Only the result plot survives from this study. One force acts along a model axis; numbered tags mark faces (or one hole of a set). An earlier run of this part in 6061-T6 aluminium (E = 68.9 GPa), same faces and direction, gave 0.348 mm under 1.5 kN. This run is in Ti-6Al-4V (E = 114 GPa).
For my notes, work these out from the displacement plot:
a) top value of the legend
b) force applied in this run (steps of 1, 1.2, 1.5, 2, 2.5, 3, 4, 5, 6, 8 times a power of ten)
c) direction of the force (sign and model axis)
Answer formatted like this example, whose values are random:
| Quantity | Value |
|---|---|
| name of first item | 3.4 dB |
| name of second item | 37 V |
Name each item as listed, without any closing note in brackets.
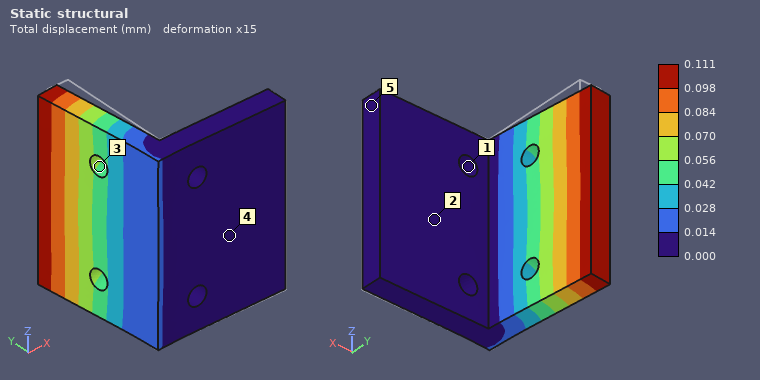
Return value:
| Quantity | Value |
|---|---|
| top value of the legend | 0.111 mm |
| force applied in this run | 800 N |
| direction of the force | -X |
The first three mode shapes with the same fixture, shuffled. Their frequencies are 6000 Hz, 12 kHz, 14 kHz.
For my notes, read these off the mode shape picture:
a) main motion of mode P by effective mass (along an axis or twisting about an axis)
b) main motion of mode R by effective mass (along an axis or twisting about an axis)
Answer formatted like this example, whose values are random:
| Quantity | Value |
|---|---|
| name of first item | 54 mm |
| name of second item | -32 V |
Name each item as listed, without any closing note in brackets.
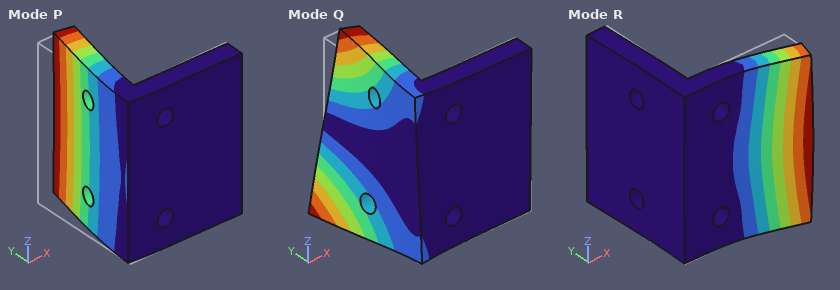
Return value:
| Quantity | Value |
|---|---|
| main motion of mode P by effective mass | along X |
| main motion of mode R by effective mass | along Y |
